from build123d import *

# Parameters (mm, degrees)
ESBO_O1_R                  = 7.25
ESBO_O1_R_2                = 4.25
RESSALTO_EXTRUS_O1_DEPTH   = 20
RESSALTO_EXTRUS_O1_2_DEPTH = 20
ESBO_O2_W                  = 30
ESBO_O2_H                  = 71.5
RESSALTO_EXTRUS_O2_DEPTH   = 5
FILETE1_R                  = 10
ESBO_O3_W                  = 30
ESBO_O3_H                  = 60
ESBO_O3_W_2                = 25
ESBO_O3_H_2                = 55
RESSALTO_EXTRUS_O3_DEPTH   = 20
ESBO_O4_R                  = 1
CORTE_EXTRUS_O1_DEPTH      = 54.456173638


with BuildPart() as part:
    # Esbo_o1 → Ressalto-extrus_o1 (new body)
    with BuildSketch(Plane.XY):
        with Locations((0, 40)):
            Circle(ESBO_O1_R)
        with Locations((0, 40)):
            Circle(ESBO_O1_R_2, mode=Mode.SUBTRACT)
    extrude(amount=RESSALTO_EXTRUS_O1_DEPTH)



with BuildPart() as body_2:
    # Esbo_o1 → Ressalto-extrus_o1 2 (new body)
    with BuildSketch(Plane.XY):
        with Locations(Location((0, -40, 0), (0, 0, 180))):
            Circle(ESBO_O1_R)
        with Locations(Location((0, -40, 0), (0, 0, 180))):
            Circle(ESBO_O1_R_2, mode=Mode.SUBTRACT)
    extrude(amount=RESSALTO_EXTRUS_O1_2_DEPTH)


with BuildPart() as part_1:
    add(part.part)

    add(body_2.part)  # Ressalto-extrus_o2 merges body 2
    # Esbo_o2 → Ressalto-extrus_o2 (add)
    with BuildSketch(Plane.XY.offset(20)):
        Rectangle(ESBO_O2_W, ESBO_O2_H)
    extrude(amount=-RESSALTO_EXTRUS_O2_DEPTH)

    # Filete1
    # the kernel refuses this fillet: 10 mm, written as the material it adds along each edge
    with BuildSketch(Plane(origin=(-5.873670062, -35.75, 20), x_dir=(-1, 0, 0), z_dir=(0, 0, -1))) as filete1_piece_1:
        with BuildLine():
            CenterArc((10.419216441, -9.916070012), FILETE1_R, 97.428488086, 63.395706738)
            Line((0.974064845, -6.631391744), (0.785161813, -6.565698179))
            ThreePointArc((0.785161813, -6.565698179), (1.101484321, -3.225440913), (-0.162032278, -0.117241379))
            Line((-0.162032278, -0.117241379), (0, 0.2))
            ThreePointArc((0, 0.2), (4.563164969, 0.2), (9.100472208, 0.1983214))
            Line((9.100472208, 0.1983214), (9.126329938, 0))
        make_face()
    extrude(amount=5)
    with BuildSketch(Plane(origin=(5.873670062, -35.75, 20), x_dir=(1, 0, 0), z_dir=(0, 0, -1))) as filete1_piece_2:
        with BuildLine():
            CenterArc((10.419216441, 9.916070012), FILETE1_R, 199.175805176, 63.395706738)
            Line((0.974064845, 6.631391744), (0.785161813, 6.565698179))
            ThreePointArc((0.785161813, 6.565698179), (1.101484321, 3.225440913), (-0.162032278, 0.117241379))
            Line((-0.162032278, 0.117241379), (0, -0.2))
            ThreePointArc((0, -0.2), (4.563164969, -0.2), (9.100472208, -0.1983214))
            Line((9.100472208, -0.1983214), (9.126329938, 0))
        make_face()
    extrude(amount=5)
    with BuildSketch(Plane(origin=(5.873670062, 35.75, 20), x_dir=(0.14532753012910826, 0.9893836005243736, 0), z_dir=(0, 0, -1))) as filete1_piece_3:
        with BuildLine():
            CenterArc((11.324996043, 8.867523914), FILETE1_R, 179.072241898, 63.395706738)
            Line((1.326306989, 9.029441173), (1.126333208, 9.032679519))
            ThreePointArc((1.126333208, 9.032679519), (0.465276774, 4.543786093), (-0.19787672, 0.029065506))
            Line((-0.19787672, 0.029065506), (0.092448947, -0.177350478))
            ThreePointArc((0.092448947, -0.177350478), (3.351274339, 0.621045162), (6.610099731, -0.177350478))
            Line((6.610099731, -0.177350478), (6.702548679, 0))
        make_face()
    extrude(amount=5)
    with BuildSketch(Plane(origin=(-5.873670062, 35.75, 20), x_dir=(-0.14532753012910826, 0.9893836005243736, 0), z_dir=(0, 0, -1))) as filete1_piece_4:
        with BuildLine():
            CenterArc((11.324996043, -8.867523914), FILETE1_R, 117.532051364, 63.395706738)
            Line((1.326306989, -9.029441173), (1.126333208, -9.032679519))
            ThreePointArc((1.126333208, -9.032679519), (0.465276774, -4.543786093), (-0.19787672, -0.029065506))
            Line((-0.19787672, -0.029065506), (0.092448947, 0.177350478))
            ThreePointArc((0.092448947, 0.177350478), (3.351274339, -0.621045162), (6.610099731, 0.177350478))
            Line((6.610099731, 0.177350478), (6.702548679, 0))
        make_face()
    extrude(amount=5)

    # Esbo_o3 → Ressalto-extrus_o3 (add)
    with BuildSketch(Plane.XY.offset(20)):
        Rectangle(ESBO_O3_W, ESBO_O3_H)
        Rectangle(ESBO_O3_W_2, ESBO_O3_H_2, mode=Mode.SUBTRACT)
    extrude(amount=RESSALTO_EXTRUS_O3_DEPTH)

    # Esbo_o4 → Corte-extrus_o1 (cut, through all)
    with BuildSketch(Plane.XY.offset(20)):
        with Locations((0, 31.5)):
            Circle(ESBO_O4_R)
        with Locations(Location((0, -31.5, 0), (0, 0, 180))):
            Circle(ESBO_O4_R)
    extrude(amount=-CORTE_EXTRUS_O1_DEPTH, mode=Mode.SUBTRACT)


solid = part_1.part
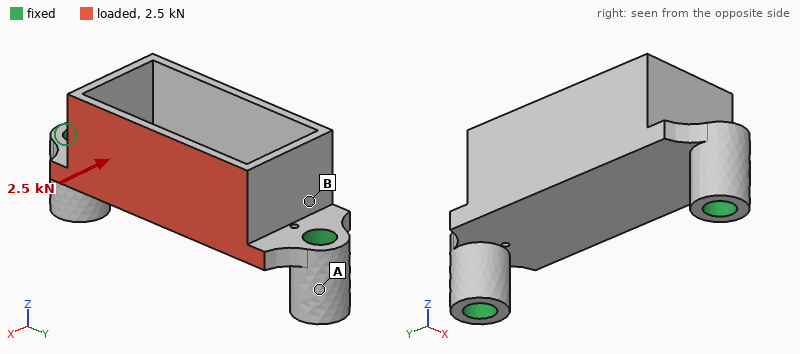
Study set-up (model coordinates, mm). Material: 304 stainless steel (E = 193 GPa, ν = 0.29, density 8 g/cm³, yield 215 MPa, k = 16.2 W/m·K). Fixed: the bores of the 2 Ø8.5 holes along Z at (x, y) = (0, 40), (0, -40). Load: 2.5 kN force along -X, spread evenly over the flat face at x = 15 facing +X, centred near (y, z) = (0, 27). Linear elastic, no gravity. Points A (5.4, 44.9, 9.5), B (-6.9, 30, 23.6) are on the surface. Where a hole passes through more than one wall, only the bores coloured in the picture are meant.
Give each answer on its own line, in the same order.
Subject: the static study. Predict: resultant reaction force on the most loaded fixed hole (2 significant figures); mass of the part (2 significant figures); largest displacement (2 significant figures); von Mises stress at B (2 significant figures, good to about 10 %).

1.3 kN
190 g
0.12 mm
39 MPa
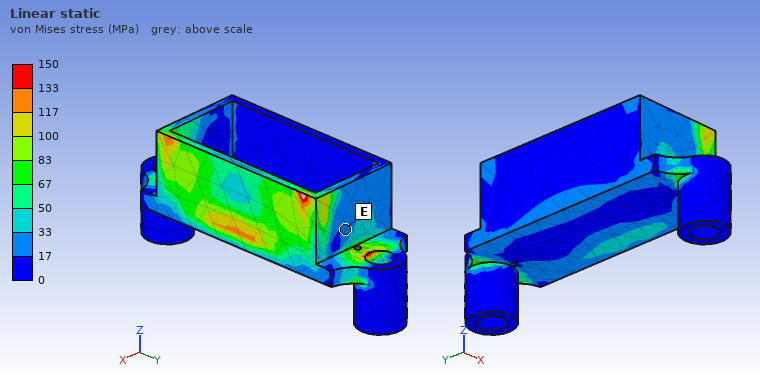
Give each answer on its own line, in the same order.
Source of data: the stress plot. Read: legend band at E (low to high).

17 to 33 MPa
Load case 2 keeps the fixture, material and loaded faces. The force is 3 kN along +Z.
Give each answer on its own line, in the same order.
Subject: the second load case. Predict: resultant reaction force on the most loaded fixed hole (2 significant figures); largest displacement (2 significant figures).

1.7 kN
75 µm
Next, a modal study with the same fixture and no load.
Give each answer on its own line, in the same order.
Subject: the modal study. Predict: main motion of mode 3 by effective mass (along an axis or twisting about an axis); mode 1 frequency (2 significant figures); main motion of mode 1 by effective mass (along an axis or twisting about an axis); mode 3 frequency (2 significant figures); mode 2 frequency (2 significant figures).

along Z
4300 Hz
along X
7500 Hz
6100 Hz
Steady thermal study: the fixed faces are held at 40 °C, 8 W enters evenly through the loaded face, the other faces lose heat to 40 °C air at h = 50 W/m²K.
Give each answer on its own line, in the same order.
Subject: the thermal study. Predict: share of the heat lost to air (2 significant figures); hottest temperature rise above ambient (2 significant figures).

65 %
33 K
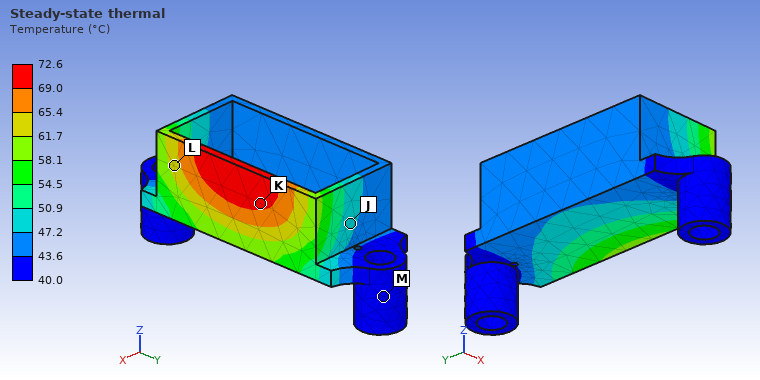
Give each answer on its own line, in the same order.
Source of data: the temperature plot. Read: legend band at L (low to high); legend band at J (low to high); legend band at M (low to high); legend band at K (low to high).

61.7 to 65.4 °C
47.2 to 50.9 °C
40.0 to 43.6 °C
69.0 to 72.6 °C
